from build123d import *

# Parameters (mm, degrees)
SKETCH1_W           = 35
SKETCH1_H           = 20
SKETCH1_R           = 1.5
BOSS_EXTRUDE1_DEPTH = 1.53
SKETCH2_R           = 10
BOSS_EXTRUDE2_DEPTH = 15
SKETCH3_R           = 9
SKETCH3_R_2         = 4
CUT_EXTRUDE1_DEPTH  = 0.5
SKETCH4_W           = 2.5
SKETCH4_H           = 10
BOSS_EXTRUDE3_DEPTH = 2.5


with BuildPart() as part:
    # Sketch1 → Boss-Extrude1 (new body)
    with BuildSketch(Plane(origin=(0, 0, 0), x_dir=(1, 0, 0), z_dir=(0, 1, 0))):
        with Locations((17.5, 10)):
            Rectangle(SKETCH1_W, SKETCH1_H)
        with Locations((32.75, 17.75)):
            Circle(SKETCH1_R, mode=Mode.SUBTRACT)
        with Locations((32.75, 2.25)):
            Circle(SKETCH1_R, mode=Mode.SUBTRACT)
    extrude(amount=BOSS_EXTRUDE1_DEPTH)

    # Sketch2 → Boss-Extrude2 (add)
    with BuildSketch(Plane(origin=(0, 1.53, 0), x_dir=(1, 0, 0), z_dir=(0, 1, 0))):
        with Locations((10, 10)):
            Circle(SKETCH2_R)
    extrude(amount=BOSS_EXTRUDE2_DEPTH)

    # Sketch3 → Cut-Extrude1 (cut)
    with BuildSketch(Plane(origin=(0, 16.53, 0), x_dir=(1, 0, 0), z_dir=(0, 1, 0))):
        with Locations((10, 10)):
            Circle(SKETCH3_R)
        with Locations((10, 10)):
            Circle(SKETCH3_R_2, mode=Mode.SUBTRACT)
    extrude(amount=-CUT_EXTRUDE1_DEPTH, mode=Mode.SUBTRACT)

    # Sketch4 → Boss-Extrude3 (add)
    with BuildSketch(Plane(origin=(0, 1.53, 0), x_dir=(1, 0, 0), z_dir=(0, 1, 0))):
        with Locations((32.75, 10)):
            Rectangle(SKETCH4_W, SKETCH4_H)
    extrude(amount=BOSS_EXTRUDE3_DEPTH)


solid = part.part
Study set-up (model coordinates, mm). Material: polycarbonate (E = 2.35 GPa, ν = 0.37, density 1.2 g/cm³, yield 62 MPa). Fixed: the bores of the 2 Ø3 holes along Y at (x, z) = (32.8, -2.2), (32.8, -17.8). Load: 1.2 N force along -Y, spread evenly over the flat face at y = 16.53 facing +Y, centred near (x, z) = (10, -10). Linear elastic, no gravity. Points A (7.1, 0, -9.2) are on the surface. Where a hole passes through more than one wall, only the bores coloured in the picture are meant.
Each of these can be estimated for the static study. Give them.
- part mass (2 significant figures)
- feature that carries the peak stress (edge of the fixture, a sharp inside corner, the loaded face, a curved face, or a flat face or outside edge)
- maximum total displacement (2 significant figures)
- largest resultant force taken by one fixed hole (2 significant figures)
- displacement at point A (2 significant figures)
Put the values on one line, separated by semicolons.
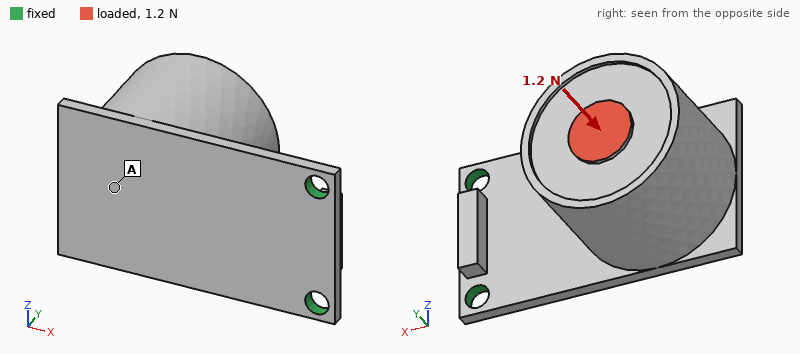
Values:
6.9 g; a flat face or outside edge; 0.52 mm; 0.61 N; 0.33 mm
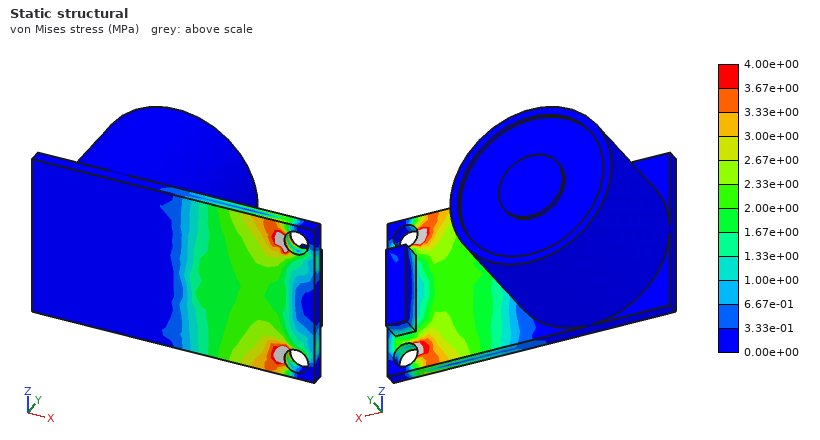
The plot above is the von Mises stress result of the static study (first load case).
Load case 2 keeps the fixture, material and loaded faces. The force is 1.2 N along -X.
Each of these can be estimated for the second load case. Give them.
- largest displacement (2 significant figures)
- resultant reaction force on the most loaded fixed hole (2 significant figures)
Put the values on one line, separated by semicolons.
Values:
0.51 mm; 0.70 N
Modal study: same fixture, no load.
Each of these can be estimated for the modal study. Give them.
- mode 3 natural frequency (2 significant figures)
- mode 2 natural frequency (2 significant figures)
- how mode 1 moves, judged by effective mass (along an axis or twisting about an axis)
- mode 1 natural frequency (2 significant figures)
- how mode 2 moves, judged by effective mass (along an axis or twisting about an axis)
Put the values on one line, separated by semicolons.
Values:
920 Hz; 370 Hz; along Y; 110 Hz; along Z
